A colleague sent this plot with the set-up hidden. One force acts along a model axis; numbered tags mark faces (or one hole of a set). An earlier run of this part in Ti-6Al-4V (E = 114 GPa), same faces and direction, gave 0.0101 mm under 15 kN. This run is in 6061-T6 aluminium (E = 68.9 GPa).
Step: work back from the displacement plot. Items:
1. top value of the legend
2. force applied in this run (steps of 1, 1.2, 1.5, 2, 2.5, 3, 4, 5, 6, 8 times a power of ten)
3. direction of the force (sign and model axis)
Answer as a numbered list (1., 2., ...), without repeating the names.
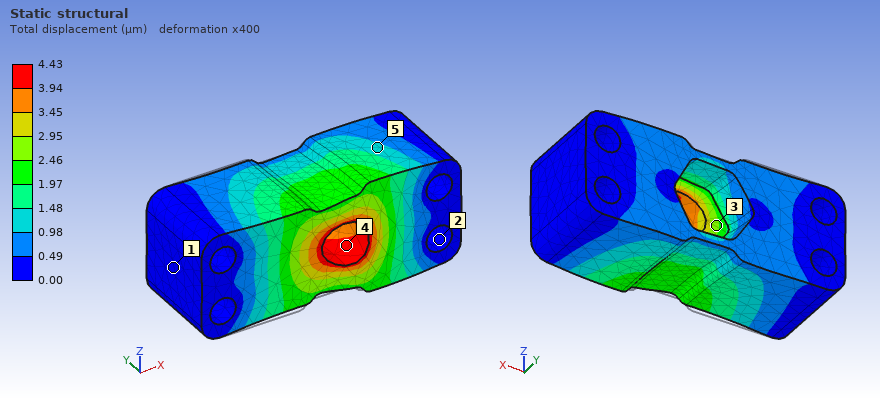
1. 4.43 µm
2. 4 kN
3. +X
